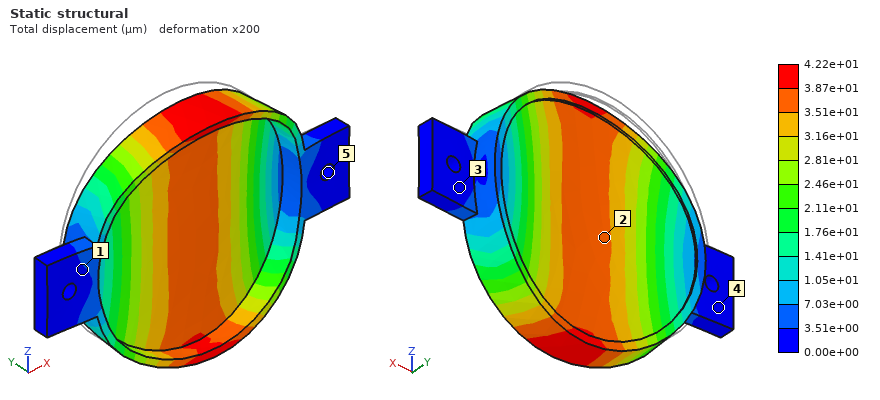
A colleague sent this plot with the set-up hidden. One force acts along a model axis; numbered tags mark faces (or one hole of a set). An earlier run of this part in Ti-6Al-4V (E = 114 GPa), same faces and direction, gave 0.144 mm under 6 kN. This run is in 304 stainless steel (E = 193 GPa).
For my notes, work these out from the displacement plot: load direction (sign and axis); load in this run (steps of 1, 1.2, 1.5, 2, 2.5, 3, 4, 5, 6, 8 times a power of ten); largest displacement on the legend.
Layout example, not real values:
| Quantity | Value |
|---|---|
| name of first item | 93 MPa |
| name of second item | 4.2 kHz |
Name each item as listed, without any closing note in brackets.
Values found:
| Quantity | Value |
|---|---|
| load direction | -Y |
| load in this run | 3 kN |
| largest displacement on the legend | 4.22e+01 µm |
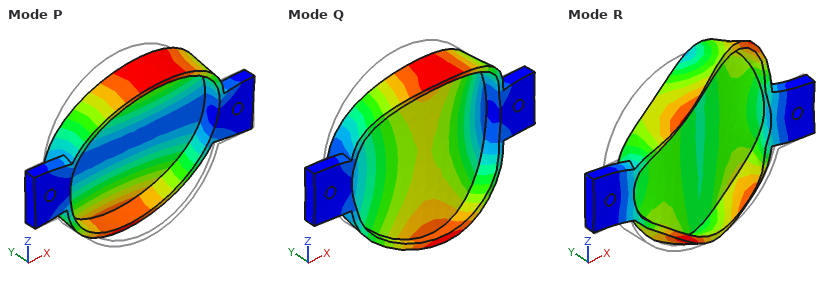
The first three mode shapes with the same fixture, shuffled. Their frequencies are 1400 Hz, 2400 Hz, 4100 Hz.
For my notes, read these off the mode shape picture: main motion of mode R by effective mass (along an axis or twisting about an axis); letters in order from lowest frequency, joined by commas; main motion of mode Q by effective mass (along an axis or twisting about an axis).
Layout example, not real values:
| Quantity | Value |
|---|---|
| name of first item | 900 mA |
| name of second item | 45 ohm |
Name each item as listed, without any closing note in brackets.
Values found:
| Quantity | Value |
|---|---|
| main motion of mode R by effective mass | along X |
| letters in order from lowest frequency, joined by commas | P, Q, R |
| main motion of mode Q by effective mass | along Y |
